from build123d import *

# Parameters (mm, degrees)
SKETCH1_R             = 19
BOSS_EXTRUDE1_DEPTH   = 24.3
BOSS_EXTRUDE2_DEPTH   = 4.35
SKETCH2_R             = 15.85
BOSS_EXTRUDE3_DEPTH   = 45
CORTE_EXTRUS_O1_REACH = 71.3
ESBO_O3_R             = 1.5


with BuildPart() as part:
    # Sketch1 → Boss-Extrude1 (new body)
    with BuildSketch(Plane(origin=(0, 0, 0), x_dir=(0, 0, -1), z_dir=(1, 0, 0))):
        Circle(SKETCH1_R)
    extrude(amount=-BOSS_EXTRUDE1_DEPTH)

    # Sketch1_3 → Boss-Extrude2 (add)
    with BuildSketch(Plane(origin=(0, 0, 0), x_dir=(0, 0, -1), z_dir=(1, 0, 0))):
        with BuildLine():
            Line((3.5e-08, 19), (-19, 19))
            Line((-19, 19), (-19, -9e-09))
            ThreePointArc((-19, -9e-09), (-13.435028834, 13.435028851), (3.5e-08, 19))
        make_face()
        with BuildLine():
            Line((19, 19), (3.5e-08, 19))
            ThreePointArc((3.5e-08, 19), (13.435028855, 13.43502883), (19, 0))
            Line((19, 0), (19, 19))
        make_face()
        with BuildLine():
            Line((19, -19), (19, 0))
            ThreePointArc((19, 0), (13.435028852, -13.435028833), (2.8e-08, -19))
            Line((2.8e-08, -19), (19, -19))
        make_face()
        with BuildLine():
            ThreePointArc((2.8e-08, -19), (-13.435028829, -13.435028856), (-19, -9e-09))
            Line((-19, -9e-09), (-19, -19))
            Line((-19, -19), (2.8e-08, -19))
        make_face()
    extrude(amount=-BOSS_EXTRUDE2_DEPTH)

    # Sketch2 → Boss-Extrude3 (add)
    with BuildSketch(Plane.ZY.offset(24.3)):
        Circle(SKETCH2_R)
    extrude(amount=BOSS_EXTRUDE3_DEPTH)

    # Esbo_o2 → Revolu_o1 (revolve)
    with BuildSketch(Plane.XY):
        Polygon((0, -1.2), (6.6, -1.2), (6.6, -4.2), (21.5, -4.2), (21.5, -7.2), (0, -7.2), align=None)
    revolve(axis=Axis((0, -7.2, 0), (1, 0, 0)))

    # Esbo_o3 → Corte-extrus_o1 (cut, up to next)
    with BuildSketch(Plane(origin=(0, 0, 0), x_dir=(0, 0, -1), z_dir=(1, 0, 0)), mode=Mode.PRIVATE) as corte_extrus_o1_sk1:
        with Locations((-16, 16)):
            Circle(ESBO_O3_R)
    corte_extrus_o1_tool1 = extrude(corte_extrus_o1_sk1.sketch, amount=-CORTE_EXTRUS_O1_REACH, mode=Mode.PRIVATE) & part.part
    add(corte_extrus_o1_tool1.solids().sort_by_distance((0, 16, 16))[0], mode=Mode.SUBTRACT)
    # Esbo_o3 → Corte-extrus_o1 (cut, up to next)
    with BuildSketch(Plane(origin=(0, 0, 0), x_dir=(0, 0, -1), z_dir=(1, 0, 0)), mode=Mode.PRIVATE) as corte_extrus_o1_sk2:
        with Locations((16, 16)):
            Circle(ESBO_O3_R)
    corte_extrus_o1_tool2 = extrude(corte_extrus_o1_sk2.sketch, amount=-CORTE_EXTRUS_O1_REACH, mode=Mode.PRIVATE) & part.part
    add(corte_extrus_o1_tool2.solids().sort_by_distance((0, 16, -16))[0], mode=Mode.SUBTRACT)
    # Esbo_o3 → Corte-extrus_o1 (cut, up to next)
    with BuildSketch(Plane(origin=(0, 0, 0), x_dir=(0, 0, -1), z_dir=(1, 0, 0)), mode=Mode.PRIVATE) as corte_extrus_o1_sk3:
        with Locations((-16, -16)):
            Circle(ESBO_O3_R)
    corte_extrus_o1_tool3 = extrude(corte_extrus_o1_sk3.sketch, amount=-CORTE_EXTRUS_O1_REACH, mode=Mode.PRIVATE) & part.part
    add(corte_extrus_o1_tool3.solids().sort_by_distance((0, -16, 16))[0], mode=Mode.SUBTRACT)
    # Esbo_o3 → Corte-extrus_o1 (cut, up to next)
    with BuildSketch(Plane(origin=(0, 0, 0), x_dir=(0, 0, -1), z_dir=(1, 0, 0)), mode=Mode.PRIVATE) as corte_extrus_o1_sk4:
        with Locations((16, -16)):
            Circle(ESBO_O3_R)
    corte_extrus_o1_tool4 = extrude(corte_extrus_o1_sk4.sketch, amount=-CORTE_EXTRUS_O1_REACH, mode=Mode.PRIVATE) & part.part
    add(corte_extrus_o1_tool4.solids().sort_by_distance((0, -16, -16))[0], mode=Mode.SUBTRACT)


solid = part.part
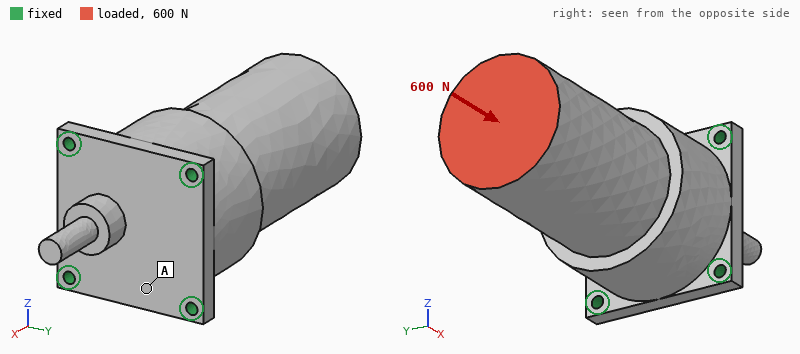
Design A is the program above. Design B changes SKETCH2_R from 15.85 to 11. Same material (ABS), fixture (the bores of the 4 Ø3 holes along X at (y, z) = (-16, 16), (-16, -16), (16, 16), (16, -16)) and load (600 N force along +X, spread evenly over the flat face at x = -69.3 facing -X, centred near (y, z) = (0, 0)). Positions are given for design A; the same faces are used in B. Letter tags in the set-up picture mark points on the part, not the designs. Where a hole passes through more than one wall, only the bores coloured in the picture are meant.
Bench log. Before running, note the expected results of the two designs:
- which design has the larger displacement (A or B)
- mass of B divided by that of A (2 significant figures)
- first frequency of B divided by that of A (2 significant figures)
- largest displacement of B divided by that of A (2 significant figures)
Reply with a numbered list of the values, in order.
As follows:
1. B
2. 0.72
3. 1.2
4. 1.3
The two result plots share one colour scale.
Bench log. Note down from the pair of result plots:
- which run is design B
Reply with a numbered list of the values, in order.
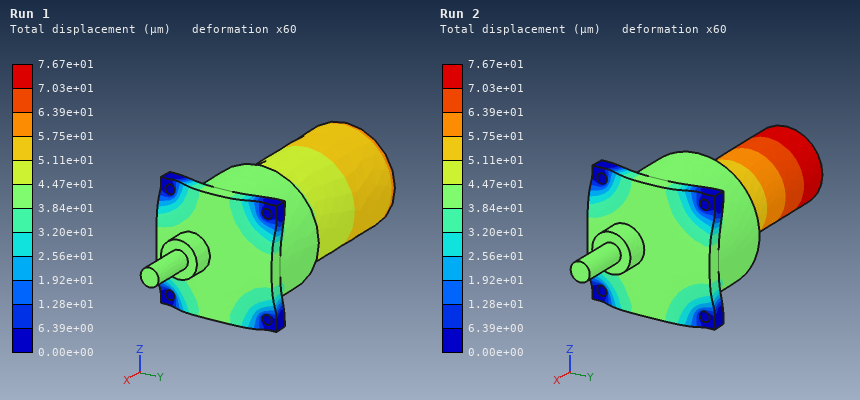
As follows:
1. Run 2
